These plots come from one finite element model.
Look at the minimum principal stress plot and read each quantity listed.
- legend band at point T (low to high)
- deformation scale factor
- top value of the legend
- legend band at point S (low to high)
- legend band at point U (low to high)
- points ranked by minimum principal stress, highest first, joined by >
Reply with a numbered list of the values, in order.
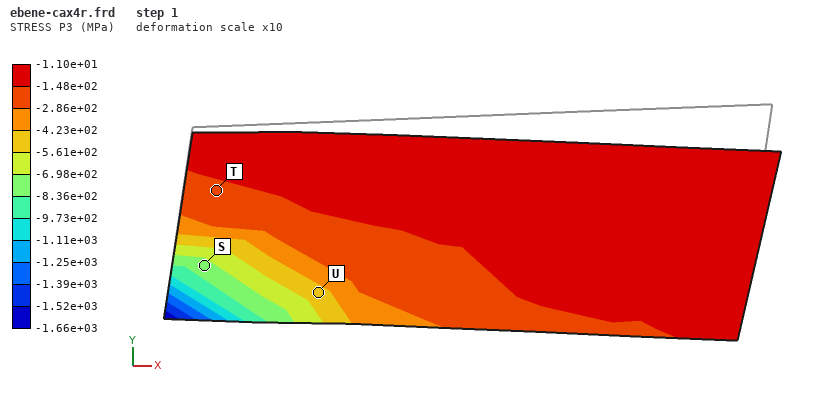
1. -2.86e+02 to -1.48e+02 MPa
2. 10
3. -1.10e+01 MPa
4. -8.36e+02 to -6.98e+02 MPa
5. -5.61e+02 to -4.23e+02 MPa
6. T > U > S
